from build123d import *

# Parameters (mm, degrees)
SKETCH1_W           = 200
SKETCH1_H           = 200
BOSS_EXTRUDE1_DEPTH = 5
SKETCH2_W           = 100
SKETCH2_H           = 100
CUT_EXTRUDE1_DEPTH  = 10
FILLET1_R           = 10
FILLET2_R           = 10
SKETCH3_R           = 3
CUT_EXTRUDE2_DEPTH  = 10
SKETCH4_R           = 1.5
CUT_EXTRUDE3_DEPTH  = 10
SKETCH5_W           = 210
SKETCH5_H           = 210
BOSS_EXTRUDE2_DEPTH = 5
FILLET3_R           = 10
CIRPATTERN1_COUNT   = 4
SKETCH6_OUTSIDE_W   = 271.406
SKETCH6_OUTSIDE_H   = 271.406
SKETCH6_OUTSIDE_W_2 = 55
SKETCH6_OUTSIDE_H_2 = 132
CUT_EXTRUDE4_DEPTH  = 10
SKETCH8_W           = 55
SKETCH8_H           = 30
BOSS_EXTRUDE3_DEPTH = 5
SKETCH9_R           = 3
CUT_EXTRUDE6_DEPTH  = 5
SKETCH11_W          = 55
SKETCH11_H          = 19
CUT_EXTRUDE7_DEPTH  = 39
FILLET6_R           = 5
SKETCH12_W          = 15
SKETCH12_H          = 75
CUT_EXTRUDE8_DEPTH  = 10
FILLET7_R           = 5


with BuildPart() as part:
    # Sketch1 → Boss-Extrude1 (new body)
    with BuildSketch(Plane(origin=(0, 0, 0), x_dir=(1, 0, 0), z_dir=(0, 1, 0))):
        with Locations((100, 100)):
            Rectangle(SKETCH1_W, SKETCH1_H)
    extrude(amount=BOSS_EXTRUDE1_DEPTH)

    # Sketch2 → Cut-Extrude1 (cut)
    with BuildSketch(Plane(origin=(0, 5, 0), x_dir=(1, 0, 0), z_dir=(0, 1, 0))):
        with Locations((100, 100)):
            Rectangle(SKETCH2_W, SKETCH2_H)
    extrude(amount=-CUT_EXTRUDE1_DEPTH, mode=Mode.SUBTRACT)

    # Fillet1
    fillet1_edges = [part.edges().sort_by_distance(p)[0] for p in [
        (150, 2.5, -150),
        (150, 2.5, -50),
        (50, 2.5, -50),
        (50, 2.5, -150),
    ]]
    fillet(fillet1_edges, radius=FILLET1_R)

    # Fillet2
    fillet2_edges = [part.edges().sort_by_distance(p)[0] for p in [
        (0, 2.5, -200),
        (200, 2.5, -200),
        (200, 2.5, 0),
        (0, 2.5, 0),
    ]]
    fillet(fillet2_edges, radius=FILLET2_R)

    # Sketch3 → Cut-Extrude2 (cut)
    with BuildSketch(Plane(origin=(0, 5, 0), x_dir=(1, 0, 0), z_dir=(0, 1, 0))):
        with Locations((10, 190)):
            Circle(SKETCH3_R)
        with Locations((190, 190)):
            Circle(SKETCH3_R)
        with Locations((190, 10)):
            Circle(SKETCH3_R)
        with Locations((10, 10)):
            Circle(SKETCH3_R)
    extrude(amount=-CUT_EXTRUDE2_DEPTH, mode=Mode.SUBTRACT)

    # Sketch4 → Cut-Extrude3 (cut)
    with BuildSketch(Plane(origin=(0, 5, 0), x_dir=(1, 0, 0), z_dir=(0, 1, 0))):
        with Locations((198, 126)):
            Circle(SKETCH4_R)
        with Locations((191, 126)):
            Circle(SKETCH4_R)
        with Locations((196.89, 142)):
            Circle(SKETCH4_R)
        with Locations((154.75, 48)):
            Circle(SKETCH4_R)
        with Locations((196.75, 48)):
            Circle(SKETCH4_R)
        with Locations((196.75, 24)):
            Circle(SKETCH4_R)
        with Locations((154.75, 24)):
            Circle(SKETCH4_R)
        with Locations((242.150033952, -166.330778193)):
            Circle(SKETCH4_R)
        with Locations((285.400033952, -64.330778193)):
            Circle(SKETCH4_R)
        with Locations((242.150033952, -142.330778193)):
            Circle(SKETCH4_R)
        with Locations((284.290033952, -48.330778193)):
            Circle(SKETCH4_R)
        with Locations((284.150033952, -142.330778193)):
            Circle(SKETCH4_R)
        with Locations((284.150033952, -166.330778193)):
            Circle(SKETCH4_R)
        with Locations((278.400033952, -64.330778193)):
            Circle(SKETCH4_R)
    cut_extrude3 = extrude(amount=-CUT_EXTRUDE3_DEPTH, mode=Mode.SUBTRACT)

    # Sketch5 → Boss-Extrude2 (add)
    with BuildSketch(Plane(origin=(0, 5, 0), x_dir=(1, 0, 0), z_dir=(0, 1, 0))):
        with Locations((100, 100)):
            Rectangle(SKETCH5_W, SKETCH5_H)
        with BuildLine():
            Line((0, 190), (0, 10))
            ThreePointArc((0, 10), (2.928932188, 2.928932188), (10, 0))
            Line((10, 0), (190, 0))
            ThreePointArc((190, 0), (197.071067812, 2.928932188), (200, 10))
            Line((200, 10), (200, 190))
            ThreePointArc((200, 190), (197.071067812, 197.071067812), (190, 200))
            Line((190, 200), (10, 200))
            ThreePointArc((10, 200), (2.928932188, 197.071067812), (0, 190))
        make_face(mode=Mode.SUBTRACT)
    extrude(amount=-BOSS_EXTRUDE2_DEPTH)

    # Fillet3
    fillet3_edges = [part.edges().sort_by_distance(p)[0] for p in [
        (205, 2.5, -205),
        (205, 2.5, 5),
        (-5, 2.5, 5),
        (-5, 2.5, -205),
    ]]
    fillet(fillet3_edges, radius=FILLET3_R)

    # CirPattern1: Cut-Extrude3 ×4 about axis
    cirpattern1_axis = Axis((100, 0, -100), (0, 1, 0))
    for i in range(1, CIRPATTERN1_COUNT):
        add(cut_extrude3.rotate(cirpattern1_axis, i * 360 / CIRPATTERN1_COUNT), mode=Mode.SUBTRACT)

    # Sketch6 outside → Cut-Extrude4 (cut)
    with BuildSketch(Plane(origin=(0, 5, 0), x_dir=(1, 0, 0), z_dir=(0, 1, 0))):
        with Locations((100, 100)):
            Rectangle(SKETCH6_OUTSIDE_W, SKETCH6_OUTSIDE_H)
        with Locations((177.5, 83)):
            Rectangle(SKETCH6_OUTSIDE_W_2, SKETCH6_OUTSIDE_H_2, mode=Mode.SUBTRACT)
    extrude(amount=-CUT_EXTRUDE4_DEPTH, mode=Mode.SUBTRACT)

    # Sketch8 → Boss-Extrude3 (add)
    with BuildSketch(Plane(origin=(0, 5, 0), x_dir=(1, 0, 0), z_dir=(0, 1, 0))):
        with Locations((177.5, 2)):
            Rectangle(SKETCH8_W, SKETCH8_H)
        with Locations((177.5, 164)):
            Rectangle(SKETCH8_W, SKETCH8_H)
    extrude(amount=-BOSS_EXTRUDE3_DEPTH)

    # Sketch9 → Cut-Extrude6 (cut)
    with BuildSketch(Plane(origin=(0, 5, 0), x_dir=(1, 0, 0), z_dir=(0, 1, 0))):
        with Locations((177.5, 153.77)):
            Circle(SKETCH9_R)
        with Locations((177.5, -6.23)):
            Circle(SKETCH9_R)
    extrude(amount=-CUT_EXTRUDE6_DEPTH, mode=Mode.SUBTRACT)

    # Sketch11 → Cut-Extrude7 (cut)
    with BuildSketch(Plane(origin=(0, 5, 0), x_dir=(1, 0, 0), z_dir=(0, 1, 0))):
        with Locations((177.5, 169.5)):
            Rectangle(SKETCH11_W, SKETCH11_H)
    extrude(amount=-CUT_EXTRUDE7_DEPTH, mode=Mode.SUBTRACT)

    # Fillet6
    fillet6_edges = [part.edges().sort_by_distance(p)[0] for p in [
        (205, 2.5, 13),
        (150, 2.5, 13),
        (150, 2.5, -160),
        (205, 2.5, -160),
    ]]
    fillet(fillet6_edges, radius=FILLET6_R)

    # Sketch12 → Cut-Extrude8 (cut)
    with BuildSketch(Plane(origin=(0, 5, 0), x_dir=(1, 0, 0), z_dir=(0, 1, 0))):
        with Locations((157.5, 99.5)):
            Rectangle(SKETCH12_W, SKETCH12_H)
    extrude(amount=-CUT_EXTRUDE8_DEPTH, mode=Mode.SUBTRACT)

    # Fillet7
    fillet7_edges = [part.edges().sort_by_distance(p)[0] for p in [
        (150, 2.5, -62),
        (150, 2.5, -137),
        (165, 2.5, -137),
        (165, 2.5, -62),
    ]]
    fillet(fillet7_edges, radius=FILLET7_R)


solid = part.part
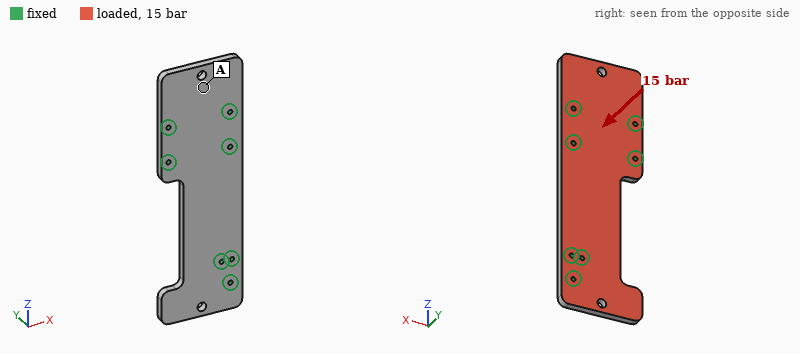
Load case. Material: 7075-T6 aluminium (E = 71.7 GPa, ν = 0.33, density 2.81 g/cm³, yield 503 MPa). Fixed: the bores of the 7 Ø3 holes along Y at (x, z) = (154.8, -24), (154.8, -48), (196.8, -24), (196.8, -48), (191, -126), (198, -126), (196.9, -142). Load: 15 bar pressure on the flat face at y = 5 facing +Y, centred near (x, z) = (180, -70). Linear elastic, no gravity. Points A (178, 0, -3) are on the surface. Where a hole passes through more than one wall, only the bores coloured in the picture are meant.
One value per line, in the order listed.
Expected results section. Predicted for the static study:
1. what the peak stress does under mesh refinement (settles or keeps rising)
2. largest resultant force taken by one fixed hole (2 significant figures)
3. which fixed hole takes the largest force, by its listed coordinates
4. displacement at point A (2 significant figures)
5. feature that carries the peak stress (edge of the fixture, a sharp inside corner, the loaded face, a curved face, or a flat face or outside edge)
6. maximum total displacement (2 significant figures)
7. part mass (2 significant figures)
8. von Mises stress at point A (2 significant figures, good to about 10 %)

keeps rising
4.4 kN
(191, -126)
0.32 mm
edge of the fixture
0.83 mm
120 g
60 MPa
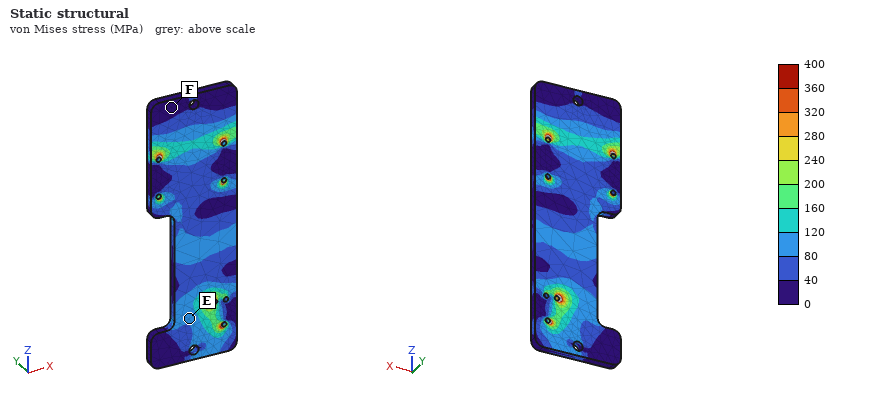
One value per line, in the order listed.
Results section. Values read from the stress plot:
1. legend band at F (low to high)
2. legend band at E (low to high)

0 to 40 MPa
80 to 120 MPa
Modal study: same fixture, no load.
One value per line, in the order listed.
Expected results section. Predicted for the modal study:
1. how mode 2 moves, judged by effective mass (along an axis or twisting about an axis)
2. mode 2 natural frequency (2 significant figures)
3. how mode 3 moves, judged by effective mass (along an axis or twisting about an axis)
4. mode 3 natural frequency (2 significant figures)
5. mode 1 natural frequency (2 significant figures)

along Y
2600 Hz
along Y
3600 Hz
2400 Hz
